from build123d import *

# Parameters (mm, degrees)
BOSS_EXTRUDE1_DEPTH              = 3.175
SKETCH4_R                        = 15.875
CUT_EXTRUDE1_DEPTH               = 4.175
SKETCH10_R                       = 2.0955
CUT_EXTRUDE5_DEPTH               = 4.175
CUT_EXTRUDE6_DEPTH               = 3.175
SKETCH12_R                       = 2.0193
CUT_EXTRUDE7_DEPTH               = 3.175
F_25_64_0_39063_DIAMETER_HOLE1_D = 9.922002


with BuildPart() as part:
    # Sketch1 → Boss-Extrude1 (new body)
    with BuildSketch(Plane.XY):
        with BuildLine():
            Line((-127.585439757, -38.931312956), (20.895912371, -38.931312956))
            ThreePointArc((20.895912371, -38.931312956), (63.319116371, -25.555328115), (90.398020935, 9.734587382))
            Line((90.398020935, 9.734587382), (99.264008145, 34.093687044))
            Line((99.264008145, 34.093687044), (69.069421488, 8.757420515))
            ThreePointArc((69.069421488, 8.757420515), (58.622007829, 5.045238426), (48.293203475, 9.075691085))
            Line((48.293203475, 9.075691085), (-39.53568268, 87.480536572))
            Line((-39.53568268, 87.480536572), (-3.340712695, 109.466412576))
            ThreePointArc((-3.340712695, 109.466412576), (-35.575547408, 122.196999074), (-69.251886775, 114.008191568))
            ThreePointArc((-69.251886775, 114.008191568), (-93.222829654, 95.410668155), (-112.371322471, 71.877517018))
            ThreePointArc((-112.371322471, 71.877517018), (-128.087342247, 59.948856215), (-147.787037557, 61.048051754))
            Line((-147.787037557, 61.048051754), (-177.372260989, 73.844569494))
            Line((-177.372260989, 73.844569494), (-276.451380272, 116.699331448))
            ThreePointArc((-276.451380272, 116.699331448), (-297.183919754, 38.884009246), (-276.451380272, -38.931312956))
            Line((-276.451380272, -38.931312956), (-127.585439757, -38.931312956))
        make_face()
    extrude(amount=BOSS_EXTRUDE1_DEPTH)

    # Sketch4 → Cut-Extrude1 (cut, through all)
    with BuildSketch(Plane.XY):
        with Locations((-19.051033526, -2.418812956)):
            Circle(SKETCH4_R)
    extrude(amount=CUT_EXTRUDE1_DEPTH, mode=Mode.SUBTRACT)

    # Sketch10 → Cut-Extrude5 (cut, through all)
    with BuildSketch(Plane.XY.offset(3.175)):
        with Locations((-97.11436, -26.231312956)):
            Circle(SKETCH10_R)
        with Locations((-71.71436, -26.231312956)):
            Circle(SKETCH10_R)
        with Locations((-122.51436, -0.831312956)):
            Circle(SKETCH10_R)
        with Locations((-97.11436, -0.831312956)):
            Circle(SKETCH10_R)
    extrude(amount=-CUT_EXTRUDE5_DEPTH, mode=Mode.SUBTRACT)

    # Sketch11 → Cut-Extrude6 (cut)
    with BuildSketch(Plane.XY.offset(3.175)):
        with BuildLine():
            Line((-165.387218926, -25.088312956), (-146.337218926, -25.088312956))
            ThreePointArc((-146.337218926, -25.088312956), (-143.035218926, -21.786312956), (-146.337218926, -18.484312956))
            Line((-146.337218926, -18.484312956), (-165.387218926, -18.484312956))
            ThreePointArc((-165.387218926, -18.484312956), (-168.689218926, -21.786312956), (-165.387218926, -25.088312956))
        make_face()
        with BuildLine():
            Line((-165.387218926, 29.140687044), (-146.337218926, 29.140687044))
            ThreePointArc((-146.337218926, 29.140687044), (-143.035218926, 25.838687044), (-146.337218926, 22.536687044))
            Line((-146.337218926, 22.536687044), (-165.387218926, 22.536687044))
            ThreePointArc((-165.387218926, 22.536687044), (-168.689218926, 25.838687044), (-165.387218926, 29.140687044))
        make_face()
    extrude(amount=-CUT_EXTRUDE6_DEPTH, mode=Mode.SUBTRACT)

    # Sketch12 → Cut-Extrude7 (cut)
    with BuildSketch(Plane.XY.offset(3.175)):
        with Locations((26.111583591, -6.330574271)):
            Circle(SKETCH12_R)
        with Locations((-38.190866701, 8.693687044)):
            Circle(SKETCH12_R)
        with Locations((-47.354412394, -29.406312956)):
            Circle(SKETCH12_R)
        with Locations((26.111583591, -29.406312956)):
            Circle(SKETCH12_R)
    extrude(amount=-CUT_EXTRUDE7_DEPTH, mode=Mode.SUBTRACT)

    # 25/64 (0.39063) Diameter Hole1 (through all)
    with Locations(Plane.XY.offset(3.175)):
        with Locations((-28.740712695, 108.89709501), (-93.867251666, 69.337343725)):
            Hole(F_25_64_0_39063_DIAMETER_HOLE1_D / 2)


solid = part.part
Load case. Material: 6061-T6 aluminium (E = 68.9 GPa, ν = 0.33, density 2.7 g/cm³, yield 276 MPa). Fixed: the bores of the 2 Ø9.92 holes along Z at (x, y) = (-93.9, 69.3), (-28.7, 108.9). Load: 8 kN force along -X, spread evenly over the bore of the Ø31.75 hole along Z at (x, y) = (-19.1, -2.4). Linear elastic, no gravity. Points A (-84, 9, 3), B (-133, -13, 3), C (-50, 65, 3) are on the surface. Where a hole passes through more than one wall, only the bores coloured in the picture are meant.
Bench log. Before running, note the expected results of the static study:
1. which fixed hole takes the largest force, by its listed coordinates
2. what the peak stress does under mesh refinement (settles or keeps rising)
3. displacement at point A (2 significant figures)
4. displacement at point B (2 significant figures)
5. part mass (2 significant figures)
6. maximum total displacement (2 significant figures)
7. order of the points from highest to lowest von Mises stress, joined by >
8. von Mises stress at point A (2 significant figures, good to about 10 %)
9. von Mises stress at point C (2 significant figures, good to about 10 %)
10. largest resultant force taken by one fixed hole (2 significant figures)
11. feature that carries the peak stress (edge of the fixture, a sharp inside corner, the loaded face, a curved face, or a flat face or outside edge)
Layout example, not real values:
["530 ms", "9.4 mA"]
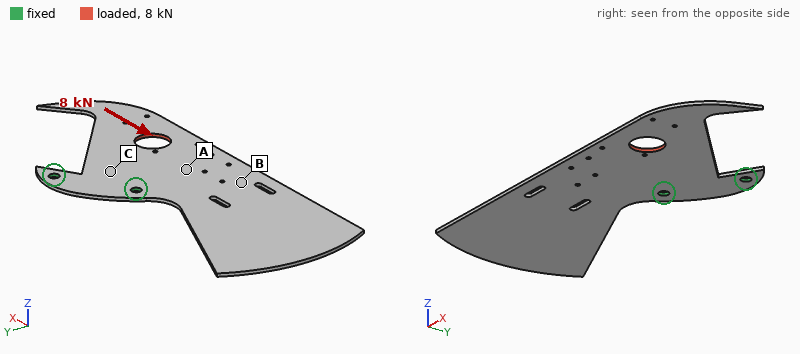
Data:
["(-93.9, 69.3)", "keeps rising", "0.30 mm", "0.46 mm", "350 g", "1.0 mm", "C > A > B", "37 MPa", "96 MPa", "12 kN", "edge of the fixture"]
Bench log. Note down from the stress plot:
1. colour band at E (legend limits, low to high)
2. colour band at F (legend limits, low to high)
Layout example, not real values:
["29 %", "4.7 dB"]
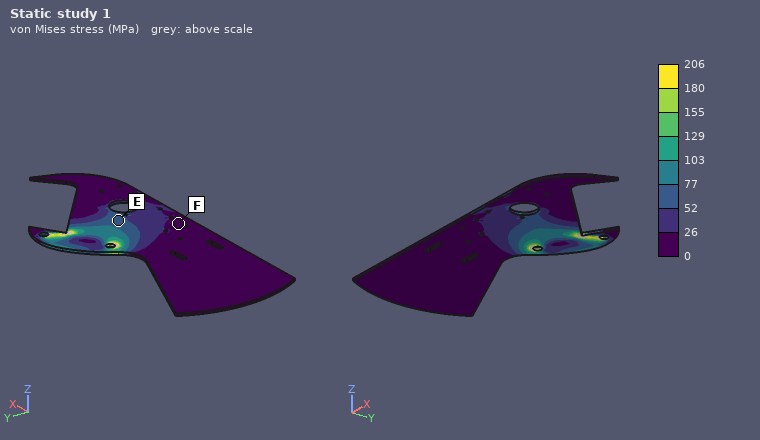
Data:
["52 to 77 MPa", "0 to 26 MPa"]
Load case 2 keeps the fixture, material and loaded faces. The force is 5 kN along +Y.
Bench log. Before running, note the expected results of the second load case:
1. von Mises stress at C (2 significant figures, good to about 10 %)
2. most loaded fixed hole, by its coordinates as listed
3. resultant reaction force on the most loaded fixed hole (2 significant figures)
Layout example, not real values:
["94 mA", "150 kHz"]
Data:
["49 MPa", "(-28.7, 108.9)", "4.8 kN"]
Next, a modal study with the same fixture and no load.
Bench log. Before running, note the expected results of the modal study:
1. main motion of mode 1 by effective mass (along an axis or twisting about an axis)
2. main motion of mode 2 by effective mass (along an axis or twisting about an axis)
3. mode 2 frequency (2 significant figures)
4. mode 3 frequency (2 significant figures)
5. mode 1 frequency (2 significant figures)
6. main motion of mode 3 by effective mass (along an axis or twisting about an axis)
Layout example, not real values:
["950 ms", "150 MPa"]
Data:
["along Z", "along Z", "100 Hz", "130 Hz", "46 Hz", "twisting about X"]
